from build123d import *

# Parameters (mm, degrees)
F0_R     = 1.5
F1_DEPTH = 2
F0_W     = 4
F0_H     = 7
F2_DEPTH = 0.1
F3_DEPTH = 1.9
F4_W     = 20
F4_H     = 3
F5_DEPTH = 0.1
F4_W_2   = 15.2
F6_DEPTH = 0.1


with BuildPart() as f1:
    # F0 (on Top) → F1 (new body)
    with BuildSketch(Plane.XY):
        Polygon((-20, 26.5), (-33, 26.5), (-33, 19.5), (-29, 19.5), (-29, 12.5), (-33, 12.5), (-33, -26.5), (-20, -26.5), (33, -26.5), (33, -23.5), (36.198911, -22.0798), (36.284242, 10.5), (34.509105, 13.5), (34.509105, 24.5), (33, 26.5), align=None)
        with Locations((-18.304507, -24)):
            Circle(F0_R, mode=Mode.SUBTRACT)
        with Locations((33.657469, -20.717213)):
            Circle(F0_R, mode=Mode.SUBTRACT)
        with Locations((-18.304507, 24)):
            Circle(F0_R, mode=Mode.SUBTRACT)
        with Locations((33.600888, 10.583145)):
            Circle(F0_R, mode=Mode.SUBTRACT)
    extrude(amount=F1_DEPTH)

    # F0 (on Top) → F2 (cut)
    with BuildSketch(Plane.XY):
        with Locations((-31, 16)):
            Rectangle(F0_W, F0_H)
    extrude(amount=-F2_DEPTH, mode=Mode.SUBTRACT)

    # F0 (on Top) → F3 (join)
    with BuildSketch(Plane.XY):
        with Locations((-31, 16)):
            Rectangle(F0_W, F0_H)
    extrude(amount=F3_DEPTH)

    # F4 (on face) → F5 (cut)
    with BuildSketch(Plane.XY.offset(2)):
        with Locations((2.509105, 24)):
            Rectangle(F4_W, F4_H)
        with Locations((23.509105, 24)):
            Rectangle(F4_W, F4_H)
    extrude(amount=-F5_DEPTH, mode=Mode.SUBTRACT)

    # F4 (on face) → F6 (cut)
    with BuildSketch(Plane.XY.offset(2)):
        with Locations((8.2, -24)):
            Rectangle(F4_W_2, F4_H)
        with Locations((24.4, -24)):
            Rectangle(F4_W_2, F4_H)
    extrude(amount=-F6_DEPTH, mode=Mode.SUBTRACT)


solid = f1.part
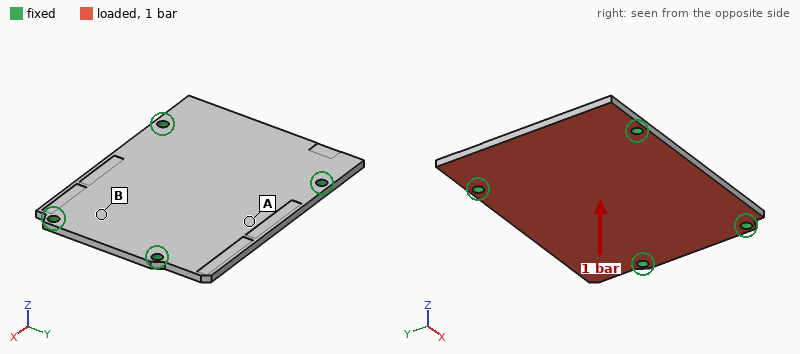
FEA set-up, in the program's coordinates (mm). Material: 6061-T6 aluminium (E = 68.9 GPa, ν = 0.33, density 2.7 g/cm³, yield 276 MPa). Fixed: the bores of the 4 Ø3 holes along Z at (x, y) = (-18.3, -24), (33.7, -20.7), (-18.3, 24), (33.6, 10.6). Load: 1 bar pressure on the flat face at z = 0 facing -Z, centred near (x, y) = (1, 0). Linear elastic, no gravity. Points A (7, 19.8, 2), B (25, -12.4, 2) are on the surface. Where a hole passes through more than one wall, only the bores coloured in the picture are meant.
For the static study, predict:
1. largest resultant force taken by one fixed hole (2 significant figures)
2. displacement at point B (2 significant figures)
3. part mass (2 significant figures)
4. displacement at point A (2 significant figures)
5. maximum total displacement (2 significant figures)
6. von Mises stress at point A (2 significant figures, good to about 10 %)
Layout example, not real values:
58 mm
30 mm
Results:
110 N
25 µm
19 g
62 µm
70 µm
22 MPa
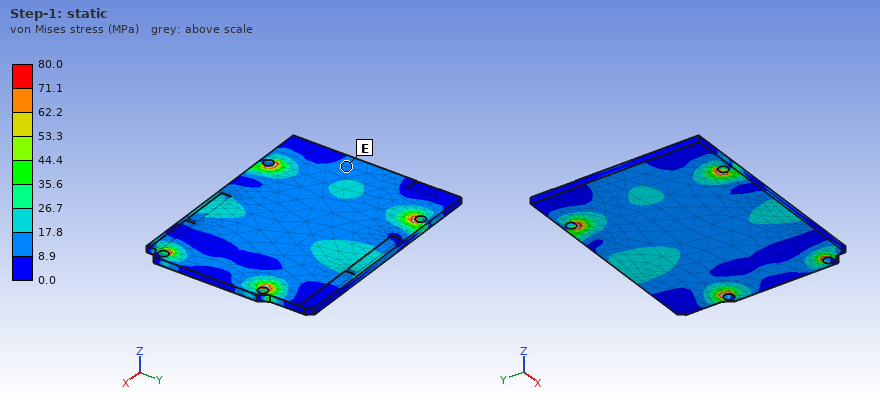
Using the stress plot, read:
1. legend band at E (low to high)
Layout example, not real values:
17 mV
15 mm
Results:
8.9 to 17.8 MPa
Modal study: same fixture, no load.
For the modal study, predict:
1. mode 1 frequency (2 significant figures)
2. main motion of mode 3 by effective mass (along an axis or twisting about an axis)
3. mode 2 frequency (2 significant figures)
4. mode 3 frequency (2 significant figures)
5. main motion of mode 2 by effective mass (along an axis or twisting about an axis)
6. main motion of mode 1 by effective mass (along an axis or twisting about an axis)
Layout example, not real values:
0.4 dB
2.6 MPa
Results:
3000 Hz
twisting about X
3700 Hz
4000 Hz
along Z
along Z
